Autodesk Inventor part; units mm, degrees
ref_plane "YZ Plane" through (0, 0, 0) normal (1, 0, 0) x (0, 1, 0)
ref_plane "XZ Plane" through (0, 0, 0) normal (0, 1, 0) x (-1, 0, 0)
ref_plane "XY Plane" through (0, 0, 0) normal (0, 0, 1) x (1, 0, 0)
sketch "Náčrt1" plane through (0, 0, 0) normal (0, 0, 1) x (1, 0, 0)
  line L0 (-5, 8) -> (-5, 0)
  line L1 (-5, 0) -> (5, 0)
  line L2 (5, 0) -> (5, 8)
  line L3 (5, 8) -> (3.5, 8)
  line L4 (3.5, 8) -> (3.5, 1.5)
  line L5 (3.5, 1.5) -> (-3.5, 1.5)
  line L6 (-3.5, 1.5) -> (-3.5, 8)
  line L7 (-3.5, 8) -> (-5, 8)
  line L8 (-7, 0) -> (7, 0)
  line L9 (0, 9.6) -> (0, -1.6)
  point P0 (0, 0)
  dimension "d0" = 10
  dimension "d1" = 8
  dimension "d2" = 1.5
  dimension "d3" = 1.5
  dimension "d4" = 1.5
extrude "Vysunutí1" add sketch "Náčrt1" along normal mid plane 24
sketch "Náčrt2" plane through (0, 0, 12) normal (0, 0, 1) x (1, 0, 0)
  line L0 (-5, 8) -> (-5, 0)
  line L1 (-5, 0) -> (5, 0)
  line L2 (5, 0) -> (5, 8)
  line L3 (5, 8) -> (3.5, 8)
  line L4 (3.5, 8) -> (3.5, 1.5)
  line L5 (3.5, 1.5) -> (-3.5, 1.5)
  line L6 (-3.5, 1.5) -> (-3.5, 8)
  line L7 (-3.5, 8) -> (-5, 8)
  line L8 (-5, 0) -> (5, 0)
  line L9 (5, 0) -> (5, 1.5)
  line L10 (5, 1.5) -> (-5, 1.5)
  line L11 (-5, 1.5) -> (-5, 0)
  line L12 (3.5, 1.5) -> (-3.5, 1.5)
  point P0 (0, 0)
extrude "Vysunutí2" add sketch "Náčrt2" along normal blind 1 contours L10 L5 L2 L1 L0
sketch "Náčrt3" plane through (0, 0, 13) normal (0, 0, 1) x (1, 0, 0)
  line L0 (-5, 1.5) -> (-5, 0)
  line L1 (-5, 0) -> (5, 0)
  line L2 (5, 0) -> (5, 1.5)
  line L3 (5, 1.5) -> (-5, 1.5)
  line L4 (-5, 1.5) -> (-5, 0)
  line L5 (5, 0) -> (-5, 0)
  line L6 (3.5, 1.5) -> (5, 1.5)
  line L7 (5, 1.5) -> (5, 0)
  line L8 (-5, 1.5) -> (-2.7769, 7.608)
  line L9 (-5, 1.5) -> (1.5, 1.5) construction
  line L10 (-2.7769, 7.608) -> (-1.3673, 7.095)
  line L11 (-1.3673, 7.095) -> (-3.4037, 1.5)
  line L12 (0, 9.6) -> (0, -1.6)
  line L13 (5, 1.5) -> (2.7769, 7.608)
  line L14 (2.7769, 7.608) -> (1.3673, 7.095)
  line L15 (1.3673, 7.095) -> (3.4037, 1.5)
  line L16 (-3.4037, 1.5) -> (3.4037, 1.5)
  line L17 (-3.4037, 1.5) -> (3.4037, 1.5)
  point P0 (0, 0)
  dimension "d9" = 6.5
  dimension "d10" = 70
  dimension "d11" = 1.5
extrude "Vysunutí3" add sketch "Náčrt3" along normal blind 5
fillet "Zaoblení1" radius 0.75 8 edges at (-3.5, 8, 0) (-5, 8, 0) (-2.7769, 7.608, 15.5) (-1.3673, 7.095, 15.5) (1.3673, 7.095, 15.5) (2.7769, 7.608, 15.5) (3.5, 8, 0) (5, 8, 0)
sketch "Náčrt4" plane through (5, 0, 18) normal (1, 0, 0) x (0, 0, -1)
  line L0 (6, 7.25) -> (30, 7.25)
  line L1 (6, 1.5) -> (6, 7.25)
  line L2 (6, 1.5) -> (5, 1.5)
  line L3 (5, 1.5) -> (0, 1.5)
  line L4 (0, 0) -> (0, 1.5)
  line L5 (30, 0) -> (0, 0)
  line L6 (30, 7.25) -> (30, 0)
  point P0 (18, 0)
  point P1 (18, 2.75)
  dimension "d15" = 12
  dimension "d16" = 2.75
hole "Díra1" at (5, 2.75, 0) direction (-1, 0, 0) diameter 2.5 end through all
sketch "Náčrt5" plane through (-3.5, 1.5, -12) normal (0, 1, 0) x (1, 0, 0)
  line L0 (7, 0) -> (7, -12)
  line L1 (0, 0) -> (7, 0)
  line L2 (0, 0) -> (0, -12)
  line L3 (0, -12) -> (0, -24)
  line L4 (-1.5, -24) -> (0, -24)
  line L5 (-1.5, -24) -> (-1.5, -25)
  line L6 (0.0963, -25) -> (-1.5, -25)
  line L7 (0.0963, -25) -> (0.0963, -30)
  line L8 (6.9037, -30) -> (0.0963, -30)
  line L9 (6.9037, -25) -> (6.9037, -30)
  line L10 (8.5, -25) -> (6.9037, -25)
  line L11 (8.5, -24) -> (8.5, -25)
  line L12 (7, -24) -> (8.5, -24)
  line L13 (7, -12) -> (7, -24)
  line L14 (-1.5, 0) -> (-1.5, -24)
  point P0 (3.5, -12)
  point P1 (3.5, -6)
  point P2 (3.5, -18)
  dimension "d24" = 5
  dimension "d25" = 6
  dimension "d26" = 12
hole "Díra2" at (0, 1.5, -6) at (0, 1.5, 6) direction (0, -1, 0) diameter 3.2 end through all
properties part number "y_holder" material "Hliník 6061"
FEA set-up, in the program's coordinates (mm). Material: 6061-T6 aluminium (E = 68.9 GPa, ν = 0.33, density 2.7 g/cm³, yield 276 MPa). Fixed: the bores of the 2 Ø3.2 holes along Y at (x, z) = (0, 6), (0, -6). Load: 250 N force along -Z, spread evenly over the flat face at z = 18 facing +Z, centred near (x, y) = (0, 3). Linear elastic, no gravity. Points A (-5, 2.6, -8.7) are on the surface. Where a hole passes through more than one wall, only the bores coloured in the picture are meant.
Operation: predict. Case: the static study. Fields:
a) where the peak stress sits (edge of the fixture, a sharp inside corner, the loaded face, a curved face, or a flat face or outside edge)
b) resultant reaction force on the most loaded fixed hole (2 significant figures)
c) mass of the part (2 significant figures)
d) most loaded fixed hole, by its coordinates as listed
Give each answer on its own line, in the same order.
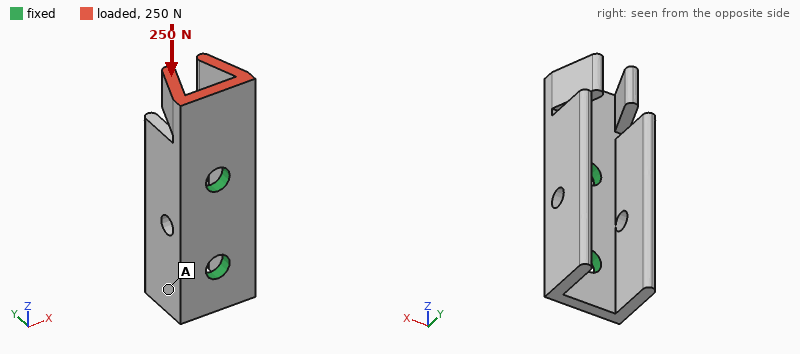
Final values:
a flat face or outside edge
180 N
2.6 g
(0, 6)
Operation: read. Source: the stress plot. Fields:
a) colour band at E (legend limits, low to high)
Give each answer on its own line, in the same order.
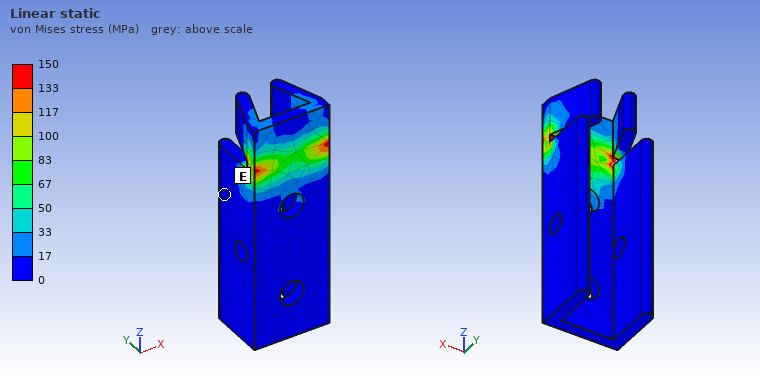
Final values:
0 to 17 MPa
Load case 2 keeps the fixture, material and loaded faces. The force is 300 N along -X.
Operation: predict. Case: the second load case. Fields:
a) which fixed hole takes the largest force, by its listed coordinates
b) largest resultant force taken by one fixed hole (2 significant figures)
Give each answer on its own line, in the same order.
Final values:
(0, 6)
450 N
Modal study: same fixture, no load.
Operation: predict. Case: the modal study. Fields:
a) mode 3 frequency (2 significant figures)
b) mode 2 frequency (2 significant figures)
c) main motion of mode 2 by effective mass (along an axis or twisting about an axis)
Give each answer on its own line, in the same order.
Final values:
15 kHz
12 kHz
along X
